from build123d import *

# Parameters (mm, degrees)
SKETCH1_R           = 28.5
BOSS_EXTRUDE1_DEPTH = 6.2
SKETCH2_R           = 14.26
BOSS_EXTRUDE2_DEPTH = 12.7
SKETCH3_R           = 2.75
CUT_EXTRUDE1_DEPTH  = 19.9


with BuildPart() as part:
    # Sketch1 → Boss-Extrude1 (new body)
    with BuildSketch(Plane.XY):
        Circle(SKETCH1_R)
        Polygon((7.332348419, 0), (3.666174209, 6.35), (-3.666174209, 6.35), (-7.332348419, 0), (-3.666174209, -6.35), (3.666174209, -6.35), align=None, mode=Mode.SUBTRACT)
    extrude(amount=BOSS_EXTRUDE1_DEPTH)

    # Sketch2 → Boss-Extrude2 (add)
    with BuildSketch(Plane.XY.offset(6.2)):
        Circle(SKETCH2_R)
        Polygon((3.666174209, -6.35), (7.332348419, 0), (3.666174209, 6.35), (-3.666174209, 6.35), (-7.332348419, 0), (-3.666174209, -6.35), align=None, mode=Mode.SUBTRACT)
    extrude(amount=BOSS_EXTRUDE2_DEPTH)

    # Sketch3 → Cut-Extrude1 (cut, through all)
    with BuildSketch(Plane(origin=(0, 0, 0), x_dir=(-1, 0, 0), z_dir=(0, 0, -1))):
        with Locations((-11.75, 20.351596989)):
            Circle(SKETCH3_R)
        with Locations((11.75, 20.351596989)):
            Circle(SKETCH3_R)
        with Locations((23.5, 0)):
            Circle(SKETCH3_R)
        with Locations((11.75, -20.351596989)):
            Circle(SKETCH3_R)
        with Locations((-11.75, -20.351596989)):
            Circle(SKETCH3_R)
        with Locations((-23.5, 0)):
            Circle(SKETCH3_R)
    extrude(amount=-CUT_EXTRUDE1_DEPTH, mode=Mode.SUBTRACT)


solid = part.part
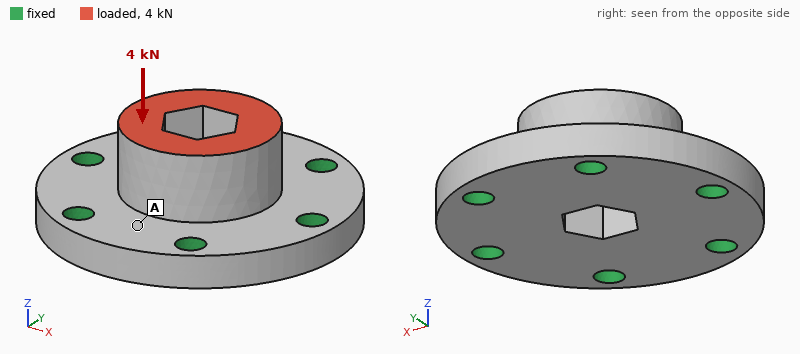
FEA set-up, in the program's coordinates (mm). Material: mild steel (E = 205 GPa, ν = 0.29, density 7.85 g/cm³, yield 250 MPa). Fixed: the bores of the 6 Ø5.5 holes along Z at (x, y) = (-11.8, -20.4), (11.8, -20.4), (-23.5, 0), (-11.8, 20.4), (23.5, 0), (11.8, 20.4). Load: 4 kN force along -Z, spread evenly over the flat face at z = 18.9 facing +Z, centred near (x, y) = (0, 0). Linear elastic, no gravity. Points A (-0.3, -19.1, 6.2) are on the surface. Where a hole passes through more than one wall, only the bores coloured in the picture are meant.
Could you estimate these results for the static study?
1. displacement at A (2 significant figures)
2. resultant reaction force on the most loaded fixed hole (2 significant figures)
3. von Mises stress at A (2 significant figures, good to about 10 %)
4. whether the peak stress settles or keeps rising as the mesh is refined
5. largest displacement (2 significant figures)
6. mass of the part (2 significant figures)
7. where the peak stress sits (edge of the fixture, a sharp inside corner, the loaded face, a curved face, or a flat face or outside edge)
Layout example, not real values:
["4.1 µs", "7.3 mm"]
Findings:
["1.00 µm", "720 N", "8.8 MPa", "keeps rising", "2.8 µm", "160 g", "edge of the fixture"]
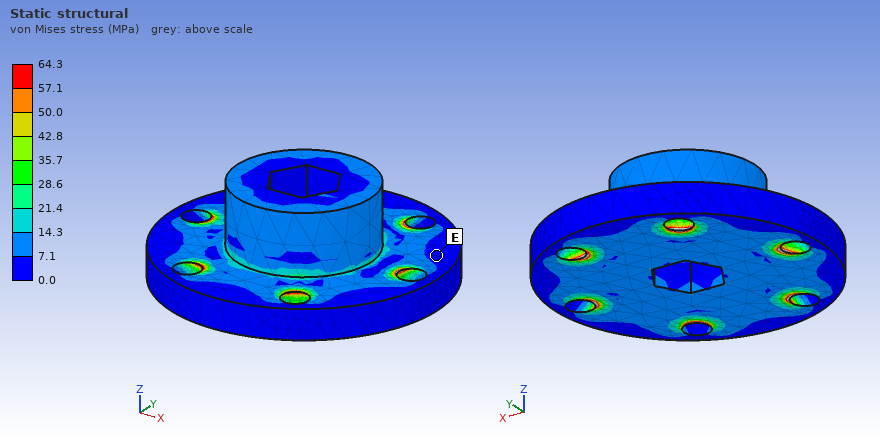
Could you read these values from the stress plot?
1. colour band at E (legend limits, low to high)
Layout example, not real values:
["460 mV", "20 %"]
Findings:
["0.0 to 7.1 MPa"]
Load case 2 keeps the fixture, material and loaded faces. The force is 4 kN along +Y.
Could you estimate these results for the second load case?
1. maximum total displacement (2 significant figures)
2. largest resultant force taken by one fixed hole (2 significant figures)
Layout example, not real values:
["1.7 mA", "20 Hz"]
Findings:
["7.4 µm", "1.3 kN"]
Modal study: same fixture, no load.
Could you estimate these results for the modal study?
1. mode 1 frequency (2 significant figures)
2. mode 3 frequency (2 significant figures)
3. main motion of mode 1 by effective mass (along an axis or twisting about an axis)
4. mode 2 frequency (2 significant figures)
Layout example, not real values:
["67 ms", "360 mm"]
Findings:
["22 kHz", "24 kHz", "along Z", "24 kHz"]
